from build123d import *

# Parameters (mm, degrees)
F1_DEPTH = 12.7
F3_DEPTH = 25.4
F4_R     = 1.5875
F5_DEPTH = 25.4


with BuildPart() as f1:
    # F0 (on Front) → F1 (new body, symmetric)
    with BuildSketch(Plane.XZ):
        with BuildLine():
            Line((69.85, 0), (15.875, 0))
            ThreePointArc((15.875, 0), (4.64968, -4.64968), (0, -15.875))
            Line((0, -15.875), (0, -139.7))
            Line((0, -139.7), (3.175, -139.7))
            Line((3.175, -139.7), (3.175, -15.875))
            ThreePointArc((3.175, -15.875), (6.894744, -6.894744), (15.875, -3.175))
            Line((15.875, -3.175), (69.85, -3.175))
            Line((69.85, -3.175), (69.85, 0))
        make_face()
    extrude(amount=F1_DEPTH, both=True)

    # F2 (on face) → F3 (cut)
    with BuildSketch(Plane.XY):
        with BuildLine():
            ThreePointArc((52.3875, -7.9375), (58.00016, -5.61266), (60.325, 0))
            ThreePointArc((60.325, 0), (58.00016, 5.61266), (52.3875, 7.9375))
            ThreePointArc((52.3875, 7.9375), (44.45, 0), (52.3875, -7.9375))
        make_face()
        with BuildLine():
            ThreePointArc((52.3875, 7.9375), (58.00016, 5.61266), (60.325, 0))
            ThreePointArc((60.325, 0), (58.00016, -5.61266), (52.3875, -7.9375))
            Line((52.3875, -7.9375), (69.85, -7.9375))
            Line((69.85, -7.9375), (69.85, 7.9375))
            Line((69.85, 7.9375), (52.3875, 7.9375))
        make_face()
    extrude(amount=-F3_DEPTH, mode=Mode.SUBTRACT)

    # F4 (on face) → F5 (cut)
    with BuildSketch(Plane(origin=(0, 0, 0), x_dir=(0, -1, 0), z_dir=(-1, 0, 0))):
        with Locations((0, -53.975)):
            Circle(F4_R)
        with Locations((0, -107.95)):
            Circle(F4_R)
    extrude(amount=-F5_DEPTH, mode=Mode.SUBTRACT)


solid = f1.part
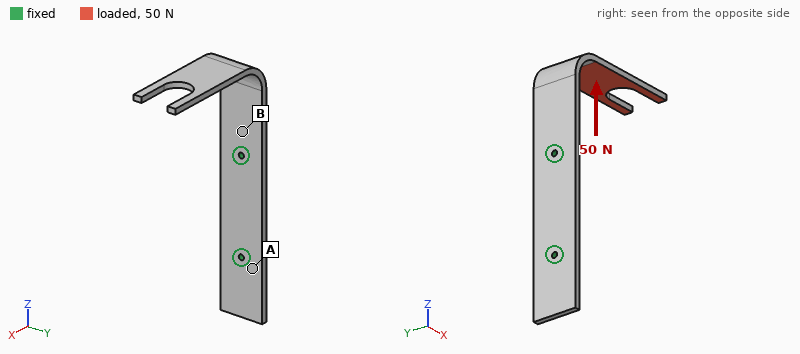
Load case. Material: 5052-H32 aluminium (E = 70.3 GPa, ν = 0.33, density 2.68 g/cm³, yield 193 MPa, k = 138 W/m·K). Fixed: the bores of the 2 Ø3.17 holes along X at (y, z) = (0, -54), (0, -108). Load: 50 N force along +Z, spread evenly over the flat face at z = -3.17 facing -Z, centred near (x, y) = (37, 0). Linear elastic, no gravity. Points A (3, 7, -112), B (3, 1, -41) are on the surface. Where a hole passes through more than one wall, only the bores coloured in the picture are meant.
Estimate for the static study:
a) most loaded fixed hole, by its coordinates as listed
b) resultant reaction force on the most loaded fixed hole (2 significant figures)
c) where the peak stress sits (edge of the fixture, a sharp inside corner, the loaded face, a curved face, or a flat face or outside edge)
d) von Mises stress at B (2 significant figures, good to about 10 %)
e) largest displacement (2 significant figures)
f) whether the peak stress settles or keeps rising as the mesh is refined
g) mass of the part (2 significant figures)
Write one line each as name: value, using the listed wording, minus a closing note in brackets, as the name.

most loaded fixed hole, by its coordinates as listed: (0, -54)
resultant reaction force on the most loaded fixed hole: 44 N
where the peak stress sits: edge of the fixture
von Mises stress at B: 40 MPa
largest displacement: 1.7 mm
whether the peak stress settles or keeps rising as the mesh is refined: keeps rising
mass of the part: 40 g
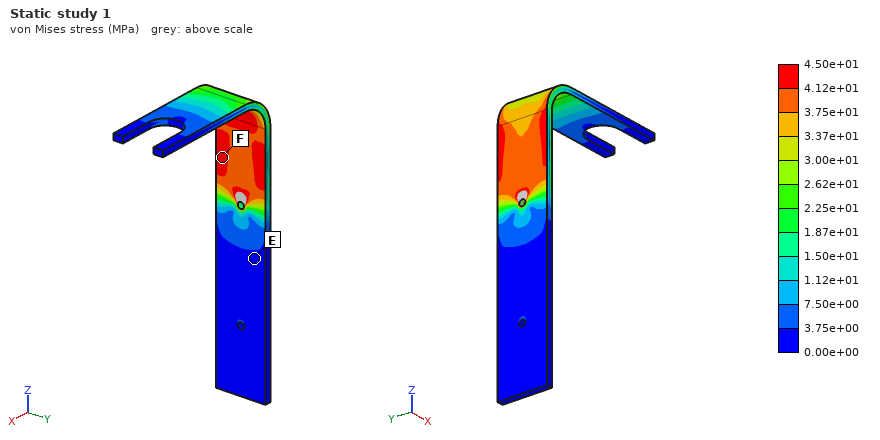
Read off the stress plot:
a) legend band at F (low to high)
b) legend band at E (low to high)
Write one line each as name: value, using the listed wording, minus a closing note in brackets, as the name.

legend band at F: 4.12e+01 to 4.50e+01 MPa
legend band at E: 0.00e+00 to 3.75e+00 MPa
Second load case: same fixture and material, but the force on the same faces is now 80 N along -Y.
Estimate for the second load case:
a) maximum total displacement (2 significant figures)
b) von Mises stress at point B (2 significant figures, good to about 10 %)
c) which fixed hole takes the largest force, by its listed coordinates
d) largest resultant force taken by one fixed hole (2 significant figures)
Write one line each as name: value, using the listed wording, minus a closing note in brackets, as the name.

maximum total displacement: 1.4 mm
von Mises stress at point B: 63 MPa
which fixed hole takes the largest force, by its listed coordinates: (0, -54)
largest resultant force taken by one fixed hole: 150 N
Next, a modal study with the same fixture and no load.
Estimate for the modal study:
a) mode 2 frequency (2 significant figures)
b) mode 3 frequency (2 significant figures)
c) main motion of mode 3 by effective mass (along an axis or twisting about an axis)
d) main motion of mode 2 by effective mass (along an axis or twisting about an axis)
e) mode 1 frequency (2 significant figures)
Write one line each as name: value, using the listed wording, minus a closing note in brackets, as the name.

mode 2 frequency: 510 Hz
mode 3 frequency: 920 Hz
main motion of mode 3 by effective mass: along X
main motion of mode 2 by effective mass: along Y
mode 1 frequency: 310 Hz
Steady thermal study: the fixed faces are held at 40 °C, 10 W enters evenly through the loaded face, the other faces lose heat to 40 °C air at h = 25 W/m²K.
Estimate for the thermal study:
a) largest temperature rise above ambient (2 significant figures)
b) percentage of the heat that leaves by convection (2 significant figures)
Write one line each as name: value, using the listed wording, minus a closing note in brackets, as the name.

largest temperature rise above ambient: 57 K
percentage of the heat that leaves by convection: 38 %
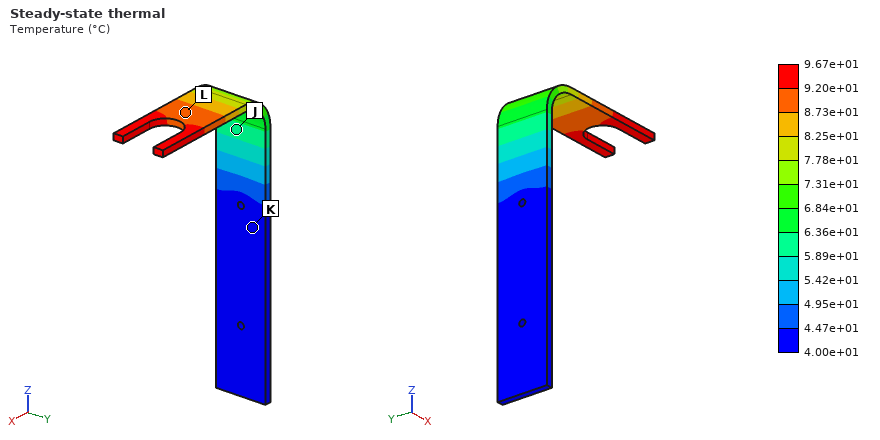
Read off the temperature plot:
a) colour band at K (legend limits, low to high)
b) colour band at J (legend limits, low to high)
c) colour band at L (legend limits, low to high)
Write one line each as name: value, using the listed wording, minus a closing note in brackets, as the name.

colour band at K: 4.00e+01 to 4.47e+01 °C
colour band at J: 5.89e+01 to 6.36e+01 °C
colour band at L: 8.73e+01 to 9.20e+01 °C
